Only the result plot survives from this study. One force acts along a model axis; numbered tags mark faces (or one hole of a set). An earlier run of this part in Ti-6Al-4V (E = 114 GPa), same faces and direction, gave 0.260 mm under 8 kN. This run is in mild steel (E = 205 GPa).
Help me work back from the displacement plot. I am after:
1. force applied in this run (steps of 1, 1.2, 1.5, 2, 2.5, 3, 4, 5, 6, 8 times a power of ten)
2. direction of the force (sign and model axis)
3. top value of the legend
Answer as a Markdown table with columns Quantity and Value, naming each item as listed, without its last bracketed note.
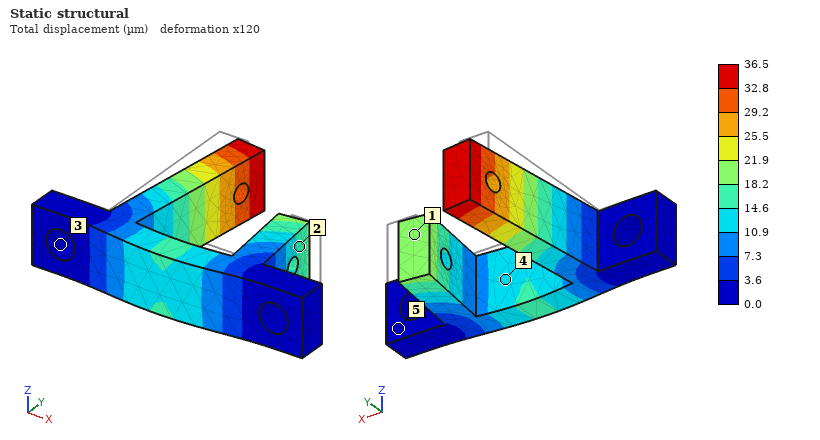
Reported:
| Quantity | Value |
|---|---|
| force applied in this run | 2 kN |
| direction of the force | -Y |
| top value of the legend | 36.5 µm |
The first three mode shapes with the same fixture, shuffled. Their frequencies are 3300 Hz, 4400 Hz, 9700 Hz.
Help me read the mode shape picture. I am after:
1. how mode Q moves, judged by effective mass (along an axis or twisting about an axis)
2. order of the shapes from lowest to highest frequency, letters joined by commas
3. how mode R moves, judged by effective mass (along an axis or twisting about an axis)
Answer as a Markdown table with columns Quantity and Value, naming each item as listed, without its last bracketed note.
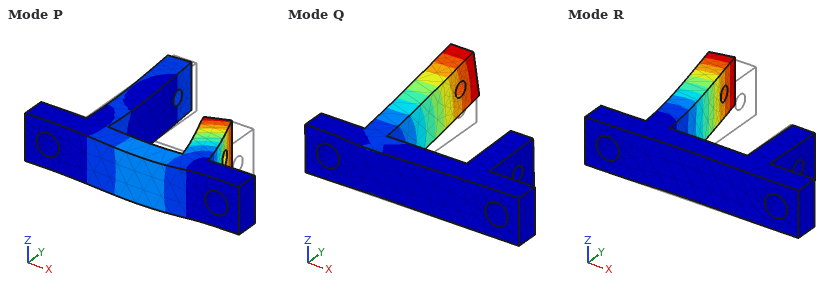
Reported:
| Quantity | Value |
|---|---|
| how mode Q moves, judged by effective mass | along Z |
| order of the shapes from lowest to highest frequency, letters joined by commas | R, Q, P |
| how mode R moves, judged by effective mass | along X |
